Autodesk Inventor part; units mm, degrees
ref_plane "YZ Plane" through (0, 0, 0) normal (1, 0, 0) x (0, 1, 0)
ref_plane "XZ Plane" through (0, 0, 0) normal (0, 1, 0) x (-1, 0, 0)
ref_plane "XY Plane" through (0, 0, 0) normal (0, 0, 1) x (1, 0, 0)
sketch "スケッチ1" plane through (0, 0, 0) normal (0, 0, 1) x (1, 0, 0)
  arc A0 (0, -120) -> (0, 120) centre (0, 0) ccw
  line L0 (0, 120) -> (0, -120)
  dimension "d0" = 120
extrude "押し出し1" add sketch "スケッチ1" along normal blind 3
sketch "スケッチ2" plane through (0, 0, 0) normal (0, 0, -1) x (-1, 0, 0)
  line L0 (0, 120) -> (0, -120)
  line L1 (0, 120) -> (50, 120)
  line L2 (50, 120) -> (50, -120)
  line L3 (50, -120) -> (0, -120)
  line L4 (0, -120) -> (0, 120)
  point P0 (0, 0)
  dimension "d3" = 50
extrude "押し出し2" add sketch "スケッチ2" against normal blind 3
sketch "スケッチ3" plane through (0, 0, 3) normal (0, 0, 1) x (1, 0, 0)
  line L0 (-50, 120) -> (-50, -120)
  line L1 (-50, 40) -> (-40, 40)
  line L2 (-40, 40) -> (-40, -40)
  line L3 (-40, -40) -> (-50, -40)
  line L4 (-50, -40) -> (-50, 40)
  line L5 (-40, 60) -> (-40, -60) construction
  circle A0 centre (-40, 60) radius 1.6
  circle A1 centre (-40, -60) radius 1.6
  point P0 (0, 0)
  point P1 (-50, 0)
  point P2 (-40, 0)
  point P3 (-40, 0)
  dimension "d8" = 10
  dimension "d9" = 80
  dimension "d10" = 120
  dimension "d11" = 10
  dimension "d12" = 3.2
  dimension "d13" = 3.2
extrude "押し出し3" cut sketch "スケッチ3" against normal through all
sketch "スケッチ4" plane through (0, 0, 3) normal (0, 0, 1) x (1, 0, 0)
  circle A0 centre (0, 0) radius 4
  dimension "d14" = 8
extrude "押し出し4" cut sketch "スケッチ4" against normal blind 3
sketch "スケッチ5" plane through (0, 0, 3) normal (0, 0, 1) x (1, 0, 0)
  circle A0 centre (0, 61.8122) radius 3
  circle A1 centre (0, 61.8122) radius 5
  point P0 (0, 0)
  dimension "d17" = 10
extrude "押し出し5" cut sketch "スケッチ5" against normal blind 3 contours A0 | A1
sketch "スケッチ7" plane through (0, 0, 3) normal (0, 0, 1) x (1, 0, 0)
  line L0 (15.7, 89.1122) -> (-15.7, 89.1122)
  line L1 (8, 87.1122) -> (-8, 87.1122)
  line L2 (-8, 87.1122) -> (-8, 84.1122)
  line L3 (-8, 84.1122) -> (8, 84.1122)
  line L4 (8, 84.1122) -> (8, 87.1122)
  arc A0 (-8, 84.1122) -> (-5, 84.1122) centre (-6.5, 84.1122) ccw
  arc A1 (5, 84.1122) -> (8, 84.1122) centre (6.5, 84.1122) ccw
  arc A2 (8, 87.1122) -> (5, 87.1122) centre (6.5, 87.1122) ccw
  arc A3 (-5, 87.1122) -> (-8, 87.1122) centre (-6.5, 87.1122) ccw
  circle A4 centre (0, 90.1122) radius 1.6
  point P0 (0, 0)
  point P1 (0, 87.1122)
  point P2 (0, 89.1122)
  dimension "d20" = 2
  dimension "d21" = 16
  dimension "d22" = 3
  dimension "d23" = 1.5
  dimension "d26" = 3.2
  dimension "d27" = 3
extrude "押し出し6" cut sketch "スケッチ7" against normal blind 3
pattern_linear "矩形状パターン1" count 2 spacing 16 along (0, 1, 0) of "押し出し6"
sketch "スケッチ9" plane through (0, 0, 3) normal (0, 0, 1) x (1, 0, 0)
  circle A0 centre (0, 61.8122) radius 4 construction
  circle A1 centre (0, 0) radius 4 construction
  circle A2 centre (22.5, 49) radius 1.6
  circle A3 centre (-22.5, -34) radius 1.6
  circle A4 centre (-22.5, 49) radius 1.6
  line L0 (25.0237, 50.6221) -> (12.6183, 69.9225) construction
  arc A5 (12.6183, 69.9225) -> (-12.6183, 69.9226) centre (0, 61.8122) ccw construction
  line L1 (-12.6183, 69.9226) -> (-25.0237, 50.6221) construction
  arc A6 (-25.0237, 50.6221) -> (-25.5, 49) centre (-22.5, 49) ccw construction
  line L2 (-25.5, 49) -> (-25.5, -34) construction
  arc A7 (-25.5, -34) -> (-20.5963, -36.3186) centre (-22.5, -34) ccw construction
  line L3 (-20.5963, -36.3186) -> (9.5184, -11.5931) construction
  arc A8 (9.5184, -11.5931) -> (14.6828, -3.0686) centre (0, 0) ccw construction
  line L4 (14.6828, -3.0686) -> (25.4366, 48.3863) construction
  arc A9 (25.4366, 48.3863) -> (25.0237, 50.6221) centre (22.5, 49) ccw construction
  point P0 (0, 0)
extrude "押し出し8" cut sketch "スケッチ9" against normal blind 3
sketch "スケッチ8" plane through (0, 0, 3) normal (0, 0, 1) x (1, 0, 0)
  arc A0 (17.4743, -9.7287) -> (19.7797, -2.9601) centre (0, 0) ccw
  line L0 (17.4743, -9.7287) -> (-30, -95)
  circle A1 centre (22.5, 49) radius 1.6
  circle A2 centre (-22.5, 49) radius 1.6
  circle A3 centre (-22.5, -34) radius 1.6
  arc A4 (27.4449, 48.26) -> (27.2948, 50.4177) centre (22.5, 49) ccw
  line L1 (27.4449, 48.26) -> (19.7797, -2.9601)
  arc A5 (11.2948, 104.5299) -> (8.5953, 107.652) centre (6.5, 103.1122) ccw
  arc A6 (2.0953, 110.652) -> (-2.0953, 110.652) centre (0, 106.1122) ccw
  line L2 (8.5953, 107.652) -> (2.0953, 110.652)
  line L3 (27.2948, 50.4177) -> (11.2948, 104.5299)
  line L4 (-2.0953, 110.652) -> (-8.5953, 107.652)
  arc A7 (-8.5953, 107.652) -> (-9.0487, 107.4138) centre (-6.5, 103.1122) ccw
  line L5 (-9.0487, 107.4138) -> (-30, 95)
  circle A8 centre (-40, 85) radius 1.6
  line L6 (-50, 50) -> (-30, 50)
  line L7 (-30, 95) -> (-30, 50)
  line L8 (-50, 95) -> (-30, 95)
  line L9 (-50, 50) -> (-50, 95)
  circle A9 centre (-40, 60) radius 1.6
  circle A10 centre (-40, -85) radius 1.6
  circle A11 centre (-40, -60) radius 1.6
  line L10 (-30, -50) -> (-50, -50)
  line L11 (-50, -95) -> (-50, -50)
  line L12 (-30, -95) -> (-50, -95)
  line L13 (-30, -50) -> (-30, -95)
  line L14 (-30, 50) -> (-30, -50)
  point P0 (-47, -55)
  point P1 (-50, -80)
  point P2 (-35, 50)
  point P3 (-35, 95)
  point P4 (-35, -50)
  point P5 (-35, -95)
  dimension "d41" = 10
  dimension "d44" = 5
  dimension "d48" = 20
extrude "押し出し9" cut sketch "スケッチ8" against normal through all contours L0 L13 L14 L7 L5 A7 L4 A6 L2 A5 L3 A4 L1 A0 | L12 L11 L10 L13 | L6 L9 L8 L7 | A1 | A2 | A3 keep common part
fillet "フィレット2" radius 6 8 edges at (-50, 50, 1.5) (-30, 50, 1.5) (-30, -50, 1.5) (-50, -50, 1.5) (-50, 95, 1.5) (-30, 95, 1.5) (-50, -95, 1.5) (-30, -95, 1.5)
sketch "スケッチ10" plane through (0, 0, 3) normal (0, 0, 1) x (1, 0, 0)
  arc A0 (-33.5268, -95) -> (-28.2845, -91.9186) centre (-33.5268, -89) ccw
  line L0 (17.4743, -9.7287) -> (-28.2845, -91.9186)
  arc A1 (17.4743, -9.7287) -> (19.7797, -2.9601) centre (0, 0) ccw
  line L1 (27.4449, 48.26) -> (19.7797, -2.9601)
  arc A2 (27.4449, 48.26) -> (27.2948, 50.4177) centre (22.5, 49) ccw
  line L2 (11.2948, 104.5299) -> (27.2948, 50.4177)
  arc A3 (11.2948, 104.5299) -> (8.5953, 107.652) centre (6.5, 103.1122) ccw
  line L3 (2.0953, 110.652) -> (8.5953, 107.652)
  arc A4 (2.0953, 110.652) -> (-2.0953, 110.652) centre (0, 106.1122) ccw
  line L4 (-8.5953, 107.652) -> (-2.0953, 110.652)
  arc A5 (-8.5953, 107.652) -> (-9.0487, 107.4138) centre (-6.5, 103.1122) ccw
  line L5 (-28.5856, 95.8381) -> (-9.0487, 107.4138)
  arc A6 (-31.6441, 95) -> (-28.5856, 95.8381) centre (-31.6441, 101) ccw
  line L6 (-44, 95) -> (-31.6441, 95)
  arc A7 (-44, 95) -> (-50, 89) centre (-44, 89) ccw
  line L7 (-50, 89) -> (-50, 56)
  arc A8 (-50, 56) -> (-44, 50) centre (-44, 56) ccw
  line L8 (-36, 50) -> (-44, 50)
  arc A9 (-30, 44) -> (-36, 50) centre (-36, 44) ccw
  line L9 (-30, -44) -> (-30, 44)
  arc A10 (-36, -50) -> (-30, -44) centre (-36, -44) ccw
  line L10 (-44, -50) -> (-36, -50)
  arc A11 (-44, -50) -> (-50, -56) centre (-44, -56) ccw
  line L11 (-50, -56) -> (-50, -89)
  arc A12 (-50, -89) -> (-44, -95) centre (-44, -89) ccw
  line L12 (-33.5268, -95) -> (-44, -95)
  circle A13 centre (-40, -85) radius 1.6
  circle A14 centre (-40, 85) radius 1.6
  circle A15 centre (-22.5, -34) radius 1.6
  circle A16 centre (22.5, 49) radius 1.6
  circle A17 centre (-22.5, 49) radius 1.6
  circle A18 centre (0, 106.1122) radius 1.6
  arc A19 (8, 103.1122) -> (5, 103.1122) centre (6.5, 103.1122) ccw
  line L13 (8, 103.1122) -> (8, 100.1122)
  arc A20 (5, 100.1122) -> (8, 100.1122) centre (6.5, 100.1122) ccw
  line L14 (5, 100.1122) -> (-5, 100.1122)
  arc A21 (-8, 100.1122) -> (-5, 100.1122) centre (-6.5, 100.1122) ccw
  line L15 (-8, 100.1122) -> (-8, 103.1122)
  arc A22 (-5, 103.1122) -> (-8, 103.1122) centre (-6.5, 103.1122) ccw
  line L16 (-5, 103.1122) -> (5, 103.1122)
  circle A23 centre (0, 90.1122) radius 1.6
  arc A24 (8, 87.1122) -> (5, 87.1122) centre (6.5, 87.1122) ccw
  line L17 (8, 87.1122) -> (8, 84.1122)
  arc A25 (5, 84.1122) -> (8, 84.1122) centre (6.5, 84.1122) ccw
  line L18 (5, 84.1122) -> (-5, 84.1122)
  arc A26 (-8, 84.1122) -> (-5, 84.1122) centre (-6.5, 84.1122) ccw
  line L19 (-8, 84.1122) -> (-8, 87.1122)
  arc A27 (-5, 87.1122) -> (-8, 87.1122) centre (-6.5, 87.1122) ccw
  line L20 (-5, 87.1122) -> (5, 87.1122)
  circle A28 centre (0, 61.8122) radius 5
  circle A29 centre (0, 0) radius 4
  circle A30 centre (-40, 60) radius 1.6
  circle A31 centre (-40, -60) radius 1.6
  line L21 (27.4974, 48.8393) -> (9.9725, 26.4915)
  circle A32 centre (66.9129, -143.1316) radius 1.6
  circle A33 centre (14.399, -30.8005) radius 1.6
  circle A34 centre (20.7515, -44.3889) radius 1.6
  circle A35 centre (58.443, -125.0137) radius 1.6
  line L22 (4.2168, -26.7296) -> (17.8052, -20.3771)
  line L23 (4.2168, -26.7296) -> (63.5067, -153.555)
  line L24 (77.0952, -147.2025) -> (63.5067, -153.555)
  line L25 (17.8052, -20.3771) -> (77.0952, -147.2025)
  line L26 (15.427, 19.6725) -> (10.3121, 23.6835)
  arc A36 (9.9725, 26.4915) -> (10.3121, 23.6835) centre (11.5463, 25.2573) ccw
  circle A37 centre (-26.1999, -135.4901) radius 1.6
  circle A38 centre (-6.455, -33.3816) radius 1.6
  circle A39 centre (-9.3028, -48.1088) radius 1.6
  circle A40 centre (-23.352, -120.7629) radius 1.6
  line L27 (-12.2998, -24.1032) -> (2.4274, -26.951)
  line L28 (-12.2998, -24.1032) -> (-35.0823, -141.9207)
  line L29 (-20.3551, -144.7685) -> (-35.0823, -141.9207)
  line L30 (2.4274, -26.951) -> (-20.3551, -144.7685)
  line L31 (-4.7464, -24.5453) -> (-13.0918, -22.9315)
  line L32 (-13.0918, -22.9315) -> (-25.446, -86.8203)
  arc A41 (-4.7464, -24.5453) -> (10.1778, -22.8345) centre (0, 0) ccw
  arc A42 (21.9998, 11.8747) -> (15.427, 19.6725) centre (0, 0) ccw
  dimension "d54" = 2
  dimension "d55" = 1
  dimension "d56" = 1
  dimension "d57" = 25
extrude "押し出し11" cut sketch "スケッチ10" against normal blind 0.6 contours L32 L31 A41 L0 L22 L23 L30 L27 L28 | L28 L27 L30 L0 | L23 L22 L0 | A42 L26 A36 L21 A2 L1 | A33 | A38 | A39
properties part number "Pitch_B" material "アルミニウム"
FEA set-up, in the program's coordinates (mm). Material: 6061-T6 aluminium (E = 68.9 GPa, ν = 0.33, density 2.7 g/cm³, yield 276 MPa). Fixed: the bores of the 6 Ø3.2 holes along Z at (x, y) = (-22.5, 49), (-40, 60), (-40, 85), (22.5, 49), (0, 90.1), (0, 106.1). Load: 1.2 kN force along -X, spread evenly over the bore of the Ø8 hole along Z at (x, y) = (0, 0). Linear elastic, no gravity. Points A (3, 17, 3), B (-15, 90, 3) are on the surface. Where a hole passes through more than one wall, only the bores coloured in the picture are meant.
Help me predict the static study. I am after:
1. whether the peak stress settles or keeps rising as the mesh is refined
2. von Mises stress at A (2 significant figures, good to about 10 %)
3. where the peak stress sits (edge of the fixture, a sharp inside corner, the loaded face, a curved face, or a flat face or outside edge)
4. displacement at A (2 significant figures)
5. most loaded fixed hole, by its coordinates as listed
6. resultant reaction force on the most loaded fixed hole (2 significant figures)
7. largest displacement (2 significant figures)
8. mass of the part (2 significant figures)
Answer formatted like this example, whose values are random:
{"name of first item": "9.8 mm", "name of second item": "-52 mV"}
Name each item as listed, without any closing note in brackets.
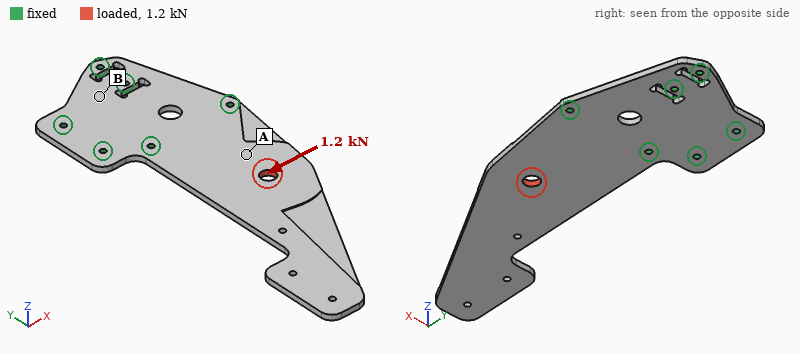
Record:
{"whether the peak stress settles or keeps rising as the mesh is refined": "keeps rising", "von Mises stress at A": "17 MPa", "where the peak stress sits": "edge of the fixture", "displacement at A": "0.023 mm", "most loaded fixed hole, by its coordinates as listed": "(22.5, 49)", "resultant reaction force on the most loaded fixed hole": "1.3 kN", "largest displacement": "0.13 mm", "mass of the part": "74 g"}
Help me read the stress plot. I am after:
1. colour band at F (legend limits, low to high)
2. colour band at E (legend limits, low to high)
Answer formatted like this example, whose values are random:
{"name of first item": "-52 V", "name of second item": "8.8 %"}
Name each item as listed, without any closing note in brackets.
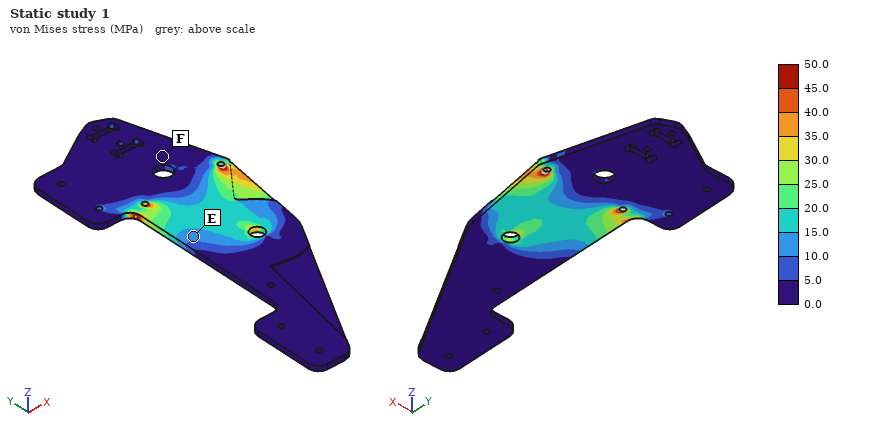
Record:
{"colour band at F": "0.0 to 5.0 MPa", "colour band at E": "10.0 to 15.0 MPa"}
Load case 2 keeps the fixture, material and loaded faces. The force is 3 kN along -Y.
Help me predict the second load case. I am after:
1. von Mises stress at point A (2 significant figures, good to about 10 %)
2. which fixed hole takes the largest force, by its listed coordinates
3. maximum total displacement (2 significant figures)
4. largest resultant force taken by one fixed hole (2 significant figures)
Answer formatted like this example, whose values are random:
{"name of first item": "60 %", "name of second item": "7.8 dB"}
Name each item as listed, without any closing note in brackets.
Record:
{"von Mises stress at point A": "29 MPa", "which fixed hole takes the largest force, by its listed coordinates": "(22.5, 49)", "maximum total displacement": "0.10 mm", "largest resultant force taken by one fixed hole": "1.4 kN"}
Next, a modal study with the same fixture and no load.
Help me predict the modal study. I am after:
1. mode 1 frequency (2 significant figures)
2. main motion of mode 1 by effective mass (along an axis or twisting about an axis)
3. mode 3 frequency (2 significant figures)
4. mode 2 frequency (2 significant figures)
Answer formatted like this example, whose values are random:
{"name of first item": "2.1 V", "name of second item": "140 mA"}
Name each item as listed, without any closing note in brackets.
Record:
{"mode 1 frequency": "140 Hz", "main motion of mode 1 by effective mass": "along Z", "mode 3 frequency": "1200 Hz", "mode 2 frequency": "620 Hz"}
